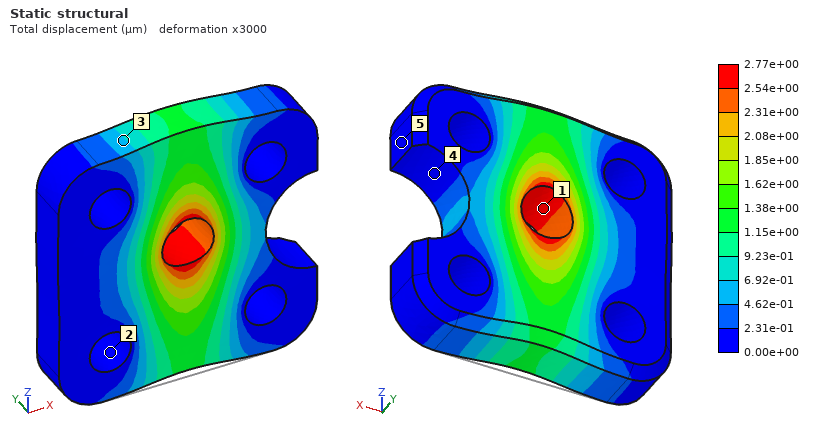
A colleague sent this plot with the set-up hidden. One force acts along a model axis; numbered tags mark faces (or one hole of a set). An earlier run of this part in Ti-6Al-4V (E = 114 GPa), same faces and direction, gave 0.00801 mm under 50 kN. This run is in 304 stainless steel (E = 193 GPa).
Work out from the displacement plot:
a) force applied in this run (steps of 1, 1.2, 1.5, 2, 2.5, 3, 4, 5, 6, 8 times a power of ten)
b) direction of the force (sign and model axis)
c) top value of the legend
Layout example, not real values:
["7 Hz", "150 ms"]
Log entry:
["30 kN", "+Z", "2.77e+00 µm"]
